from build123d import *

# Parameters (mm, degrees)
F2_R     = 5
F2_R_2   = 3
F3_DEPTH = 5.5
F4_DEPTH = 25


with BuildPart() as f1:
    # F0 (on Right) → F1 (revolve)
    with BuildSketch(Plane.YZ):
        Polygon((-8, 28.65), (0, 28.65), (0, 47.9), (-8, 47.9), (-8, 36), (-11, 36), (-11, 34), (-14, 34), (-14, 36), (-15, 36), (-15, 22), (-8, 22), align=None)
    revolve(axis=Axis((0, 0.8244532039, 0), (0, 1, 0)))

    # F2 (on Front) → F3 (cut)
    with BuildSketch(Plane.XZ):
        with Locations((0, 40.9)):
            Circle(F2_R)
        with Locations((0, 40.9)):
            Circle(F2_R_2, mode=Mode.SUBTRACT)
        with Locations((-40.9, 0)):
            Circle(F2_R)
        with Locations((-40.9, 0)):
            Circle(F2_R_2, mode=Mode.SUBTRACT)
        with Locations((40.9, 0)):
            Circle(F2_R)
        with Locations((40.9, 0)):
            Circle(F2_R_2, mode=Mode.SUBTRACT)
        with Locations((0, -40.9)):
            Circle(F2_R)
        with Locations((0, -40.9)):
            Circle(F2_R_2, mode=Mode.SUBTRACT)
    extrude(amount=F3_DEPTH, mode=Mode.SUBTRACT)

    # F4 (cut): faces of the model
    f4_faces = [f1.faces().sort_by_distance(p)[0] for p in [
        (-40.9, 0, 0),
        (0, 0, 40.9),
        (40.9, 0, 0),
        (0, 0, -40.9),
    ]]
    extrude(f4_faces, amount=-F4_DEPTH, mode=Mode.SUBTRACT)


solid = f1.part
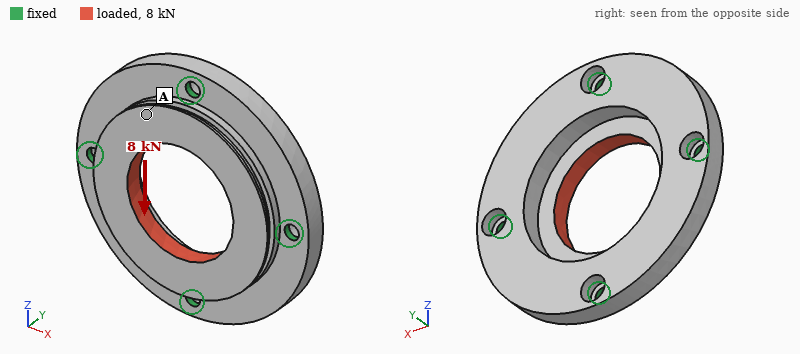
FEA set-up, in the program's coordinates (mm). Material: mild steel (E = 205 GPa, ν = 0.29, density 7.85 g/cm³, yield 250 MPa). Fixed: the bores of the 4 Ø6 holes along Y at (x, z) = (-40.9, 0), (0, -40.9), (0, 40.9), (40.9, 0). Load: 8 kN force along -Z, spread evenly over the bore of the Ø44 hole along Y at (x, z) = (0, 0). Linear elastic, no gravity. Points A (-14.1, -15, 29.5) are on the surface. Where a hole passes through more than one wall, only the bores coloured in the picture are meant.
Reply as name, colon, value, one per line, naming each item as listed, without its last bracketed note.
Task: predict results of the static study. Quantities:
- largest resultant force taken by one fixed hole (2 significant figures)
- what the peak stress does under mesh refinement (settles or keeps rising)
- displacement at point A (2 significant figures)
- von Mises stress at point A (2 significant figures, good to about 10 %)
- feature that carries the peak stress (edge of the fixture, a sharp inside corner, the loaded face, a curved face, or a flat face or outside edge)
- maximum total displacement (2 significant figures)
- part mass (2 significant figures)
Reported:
largest resultant force taken by one fixed hole: 2.1 kN
what the peak stress does under mesh refinement: keeps rising
displacement at point A: 3.5 µm
von Mises stress at point A: 11 MPa
feature that carries the peak stress: edge of the fixture
maximum total displacement: 4.3 µm
part mass: 400 g
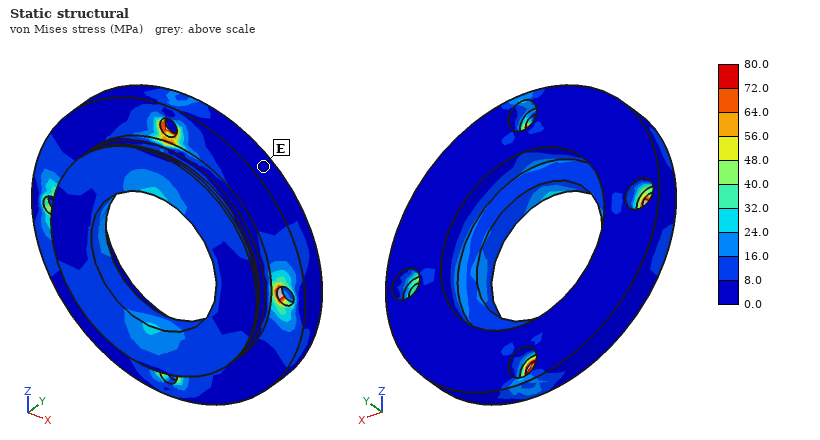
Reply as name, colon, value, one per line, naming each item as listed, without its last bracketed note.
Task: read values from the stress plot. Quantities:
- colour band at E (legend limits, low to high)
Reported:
colour band at E: 0.0 to 8.0 MPa
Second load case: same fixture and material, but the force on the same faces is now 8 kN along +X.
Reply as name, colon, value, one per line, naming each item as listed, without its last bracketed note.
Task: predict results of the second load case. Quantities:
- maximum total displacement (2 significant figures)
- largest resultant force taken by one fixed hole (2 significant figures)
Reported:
maximum total displacement: 4.3 µm
largest resultant force taken by one fixed hole: 2.1 kN
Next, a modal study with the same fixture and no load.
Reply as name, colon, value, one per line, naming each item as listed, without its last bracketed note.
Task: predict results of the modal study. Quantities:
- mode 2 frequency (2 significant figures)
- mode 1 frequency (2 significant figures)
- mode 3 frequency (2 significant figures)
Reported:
mode 2 frequency: 8100 Hz
mode 1 frequency: 6000 Hz
mode 3 frequency: 8100 Hz
